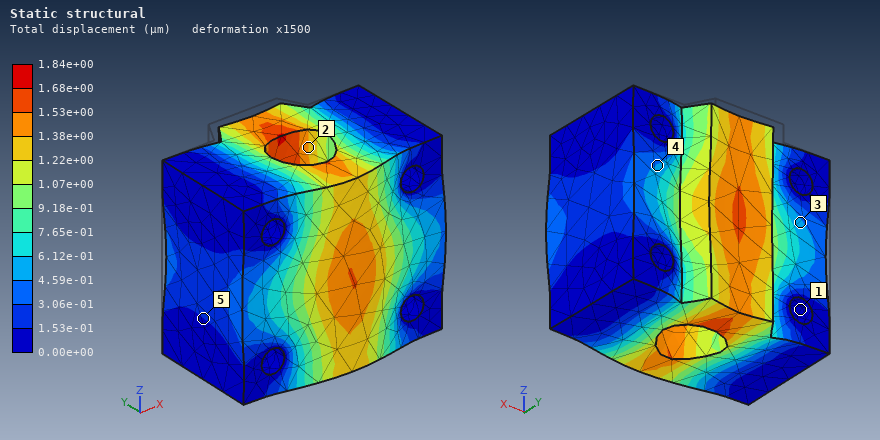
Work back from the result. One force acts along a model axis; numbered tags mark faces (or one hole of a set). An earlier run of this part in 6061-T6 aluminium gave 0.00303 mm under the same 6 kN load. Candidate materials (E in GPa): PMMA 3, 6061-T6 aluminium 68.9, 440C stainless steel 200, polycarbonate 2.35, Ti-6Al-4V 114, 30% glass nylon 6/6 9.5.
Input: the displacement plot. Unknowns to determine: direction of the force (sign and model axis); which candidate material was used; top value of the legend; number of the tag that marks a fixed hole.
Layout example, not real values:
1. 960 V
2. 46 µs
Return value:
1. -Y
2. Ti-6Al-4V
3. 1.84e+00 µm
4. 1
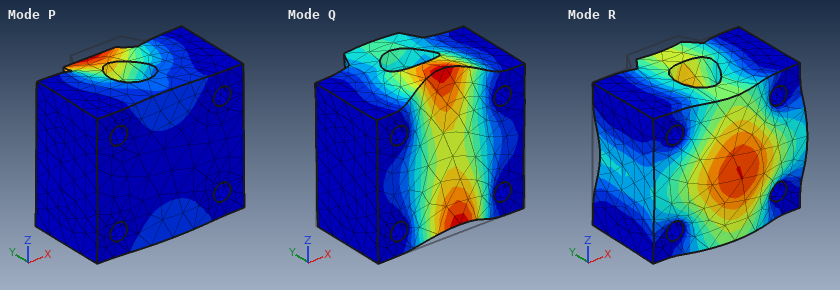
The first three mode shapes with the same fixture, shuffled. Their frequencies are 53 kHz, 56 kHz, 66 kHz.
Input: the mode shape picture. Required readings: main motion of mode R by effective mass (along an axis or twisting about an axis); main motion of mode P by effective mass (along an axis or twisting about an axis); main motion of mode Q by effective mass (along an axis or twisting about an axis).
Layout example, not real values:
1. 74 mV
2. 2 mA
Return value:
1. along Y
2. along Z
3. along Z
